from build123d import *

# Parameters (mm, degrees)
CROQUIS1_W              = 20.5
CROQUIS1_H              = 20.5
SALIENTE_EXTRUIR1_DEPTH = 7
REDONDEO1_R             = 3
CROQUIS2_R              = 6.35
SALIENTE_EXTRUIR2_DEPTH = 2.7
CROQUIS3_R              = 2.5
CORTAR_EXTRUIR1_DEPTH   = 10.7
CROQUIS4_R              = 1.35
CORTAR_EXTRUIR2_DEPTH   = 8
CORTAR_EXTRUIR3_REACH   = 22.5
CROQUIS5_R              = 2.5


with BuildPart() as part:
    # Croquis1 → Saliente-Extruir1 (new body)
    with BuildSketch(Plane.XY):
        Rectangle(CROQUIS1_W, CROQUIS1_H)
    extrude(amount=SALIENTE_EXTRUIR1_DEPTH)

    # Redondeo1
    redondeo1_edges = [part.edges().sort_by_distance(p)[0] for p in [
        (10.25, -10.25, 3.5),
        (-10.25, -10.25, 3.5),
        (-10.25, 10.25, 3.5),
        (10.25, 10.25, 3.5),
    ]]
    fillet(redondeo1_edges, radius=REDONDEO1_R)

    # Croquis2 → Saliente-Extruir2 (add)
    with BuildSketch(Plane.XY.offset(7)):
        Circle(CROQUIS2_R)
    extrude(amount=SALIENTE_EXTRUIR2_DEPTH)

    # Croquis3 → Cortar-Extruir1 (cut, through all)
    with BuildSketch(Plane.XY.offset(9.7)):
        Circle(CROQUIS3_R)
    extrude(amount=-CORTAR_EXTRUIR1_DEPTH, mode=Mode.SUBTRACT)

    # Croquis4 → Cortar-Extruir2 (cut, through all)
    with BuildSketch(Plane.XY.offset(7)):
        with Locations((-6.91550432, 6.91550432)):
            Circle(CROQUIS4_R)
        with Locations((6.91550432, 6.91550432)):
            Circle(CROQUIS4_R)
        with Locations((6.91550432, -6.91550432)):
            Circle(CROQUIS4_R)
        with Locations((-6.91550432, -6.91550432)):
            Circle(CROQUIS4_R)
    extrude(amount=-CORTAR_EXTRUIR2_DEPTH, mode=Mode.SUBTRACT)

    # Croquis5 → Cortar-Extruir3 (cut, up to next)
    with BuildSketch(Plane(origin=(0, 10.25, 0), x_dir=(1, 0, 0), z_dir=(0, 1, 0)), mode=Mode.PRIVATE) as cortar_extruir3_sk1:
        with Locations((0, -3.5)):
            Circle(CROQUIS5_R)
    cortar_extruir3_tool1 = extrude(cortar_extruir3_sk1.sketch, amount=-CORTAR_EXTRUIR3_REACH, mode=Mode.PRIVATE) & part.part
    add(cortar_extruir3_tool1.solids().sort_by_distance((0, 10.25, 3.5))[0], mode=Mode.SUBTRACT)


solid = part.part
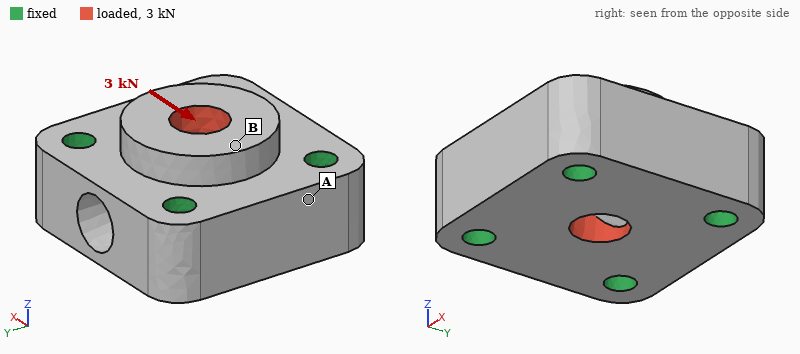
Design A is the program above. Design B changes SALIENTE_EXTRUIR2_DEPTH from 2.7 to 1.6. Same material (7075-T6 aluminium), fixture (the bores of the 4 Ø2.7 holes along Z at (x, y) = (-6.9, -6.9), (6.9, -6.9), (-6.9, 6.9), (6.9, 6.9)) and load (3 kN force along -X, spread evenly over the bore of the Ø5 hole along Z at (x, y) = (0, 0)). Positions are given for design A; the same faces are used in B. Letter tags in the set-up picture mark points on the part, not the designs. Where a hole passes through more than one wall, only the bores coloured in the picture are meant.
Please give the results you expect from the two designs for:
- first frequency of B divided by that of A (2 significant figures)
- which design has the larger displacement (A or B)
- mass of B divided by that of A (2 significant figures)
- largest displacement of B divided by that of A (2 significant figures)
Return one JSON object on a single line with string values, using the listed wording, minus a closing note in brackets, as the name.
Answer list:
{"first frequency of B divided by that of A": "1.0", "which design has the larger displacement": "A", "mass of B divided by that of A": "0.96", "largest displacement of B divided by that of A": "0.89"}
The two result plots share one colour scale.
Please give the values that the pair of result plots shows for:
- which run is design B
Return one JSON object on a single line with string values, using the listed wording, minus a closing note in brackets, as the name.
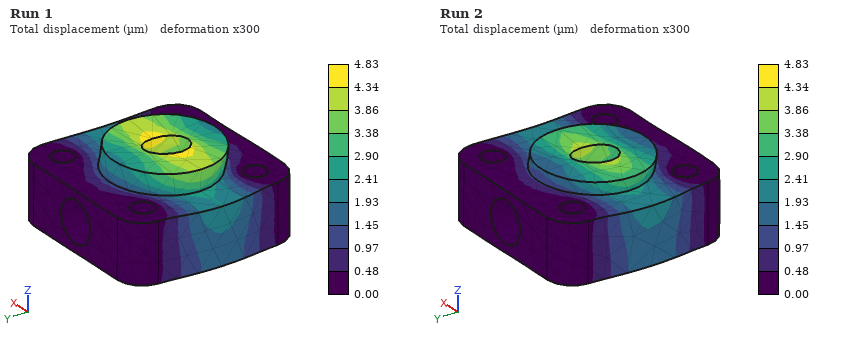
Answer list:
{"which run is design B": "Run 2"}
